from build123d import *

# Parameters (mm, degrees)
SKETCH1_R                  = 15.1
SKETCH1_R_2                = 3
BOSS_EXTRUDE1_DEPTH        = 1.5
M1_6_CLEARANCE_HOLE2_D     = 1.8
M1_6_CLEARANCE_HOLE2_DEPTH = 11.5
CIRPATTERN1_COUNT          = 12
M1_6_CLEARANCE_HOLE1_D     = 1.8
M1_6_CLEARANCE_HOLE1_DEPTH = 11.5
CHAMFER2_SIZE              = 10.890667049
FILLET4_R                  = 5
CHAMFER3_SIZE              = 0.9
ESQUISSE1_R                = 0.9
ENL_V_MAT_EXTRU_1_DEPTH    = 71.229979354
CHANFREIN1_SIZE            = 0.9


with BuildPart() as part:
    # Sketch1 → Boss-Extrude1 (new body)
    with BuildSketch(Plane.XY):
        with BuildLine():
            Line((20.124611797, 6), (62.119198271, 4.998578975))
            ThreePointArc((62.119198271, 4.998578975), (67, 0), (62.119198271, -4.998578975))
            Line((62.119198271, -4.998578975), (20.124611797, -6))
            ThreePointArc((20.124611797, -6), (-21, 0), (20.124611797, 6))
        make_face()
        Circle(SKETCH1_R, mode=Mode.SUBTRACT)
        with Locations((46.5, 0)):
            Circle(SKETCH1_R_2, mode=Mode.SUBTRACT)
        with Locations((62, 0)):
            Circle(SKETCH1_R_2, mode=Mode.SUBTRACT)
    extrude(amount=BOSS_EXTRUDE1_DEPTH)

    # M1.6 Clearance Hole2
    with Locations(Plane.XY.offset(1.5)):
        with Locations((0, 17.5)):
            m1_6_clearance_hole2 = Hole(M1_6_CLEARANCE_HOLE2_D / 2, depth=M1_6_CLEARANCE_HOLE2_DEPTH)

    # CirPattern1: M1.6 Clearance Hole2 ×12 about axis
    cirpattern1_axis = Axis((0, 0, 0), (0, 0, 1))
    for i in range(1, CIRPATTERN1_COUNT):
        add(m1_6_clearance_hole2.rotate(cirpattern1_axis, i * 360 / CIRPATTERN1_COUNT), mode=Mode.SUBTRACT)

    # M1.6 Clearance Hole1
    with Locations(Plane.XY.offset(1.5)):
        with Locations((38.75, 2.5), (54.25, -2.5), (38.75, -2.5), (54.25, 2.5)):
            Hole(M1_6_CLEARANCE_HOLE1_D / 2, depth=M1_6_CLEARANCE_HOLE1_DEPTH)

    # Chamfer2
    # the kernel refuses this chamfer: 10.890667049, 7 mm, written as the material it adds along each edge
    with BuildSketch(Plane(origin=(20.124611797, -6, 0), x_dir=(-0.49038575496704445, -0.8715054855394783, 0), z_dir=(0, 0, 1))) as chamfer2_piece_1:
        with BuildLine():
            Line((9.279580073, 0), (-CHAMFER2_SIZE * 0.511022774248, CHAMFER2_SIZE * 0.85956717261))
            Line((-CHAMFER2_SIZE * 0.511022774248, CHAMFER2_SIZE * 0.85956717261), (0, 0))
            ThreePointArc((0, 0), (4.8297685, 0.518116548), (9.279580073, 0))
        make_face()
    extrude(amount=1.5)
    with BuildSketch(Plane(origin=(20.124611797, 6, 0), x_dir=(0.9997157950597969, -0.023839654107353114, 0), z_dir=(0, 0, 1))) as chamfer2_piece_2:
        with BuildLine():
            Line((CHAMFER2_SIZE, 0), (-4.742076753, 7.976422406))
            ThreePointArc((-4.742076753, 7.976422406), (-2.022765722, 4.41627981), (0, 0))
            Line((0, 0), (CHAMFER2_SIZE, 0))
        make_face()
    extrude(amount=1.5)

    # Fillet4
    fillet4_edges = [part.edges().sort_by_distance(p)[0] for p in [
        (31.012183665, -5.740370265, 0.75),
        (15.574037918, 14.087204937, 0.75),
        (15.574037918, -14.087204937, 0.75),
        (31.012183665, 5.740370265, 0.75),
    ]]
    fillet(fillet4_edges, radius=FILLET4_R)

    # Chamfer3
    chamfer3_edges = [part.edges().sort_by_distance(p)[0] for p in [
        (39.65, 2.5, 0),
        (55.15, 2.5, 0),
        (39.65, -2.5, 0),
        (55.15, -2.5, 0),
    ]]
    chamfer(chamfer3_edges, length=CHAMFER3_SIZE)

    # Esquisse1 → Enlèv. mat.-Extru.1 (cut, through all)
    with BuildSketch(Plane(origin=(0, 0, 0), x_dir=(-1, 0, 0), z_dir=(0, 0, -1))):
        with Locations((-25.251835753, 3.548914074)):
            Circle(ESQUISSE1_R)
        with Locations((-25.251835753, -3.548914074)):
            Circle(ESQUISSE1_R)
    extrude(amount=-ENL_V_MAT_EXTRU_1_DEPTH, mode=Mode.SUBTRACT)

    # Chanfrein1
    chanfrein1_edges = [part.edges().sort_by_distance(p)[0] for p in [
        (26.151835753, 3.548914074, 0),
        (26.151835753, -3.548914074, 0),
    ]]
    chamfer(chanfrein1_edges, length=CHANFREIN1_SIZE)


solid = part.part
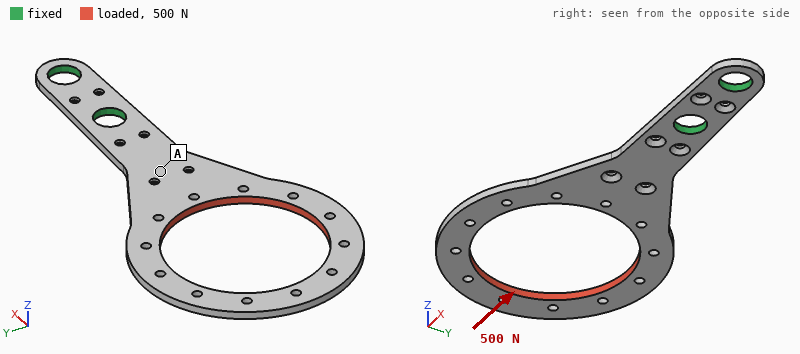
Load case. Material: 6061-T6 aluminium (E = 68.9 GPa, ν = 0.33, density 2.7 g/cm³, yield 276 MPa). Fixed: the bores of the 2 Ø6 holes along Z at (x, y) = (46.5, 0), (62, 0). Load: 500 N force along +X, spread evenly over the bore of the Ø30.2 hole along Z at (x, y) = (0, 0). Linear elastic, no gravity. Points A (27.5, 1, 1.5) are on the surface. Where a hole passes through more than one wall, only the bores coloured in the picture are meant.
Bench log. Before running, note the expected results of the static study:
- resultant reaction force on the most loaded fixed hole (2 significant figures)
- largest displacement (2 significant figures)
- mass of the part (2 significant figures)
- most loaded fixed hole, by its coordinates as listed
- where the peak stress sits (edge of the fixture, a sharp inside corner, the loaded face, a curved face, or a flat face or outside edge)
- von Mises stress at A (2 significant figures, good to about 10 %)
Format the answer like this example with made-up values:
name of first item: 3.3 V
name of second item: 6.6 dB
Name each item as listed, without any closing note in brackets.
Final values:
resultant reaction force on the most loaded fixed hole: 490 N
largest displacement: 0.12 mm
mass of the part: 4.6 g
most loaded fixed hole, by its coordinates as listed: (46.5, 0)
where the peak stress sits: a curved face
von Mises stress at A: 14 MPa
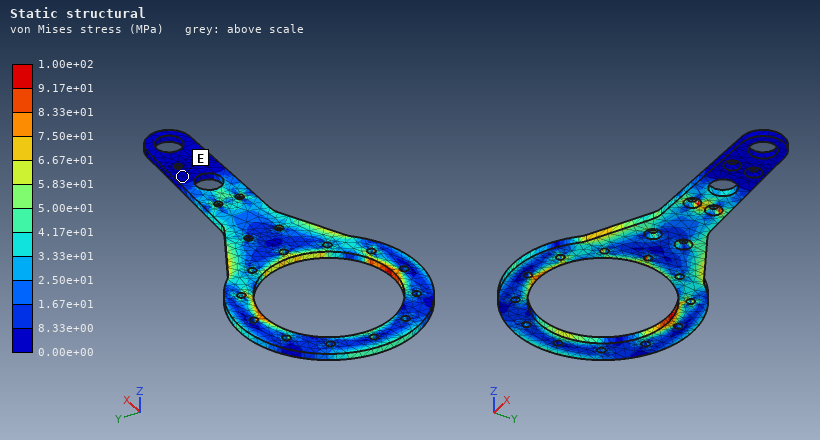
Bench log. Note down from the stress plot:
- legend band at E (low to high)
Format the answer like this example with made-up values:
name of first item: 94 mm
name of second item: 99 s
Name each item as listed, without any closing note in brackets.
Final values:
legend band at E: 0.00e+00 to 8.33e+00 MPa
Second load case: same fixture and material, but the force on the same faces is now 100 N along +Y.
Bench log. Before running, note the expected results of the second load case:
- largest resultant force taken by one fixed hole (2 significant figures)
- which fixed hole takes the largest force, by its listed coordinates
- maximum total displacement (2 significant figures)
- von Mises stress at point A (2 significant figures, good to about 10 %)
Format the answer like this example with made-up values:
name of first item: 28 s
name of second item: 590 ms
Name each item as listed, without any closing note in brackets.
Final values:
largest resultant force taken by one fixed hole: 130 N
which fixed hole takes the largest force, by its listed coordinates: (46.5, 0)
maximum total displacement: 0.50 mm
von Mises stress at point A: 28 MPa
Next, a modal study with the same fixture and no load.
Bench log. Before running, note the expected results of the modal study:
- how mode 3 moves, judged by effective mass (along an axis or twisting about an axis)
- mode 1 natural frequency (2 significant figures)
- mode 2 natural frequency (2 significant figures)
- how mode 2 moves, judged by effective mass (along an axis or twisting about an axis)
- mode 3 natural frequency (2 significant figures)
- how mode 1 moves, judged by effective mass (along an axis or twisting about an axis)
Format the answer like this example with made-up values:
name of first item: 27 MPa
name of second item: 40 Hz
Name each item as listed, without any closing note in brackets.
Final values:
how mode 3 moves, judged by effective mass: along Z
mode 1 natural frequency: 240 Hz
mode 2 natural frequency: 710 Hz
how mode 2 moves, judged by effective mass: twisting about X
mode 3 natural frequency: 1400 Hz
how mode 1 moves, judged by effective mass: along Z
